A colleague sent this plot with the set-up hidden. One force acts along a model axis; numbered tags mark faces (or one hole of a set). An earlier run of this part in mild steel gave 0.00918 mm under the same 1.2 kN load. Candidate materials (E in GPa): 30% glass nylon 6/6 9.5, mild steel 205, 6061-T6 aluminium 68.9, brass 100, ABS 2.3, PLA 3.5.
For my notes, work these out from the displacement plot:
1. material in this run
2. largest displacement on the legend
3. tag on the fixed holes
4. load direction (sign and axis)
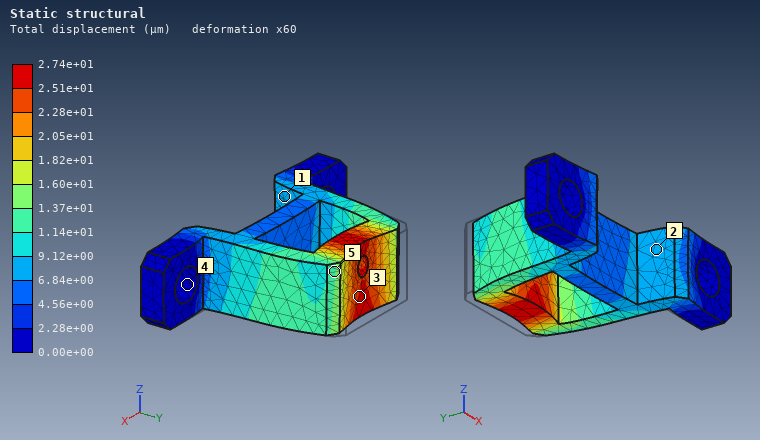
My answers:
6061-T6 aluminium
2.74e+01 µm
4
-Y
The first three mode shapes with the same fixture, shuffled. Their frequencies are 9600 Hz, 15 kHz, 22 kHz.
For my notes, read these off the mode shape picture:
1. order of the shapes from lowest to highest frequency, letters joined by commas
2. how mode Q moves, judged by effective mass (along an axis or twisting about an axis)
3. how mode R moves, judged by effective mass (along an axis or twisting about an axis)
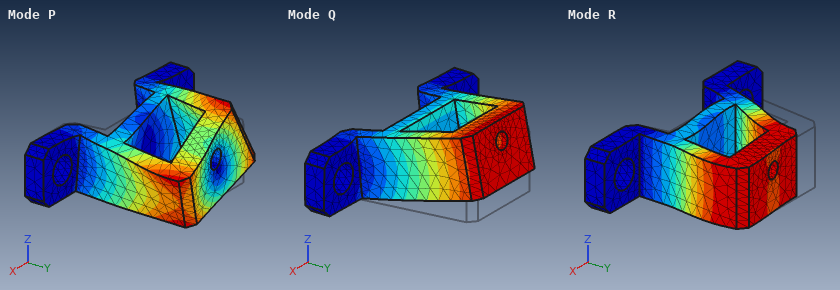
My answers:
Q, R, P
along Z
along X
